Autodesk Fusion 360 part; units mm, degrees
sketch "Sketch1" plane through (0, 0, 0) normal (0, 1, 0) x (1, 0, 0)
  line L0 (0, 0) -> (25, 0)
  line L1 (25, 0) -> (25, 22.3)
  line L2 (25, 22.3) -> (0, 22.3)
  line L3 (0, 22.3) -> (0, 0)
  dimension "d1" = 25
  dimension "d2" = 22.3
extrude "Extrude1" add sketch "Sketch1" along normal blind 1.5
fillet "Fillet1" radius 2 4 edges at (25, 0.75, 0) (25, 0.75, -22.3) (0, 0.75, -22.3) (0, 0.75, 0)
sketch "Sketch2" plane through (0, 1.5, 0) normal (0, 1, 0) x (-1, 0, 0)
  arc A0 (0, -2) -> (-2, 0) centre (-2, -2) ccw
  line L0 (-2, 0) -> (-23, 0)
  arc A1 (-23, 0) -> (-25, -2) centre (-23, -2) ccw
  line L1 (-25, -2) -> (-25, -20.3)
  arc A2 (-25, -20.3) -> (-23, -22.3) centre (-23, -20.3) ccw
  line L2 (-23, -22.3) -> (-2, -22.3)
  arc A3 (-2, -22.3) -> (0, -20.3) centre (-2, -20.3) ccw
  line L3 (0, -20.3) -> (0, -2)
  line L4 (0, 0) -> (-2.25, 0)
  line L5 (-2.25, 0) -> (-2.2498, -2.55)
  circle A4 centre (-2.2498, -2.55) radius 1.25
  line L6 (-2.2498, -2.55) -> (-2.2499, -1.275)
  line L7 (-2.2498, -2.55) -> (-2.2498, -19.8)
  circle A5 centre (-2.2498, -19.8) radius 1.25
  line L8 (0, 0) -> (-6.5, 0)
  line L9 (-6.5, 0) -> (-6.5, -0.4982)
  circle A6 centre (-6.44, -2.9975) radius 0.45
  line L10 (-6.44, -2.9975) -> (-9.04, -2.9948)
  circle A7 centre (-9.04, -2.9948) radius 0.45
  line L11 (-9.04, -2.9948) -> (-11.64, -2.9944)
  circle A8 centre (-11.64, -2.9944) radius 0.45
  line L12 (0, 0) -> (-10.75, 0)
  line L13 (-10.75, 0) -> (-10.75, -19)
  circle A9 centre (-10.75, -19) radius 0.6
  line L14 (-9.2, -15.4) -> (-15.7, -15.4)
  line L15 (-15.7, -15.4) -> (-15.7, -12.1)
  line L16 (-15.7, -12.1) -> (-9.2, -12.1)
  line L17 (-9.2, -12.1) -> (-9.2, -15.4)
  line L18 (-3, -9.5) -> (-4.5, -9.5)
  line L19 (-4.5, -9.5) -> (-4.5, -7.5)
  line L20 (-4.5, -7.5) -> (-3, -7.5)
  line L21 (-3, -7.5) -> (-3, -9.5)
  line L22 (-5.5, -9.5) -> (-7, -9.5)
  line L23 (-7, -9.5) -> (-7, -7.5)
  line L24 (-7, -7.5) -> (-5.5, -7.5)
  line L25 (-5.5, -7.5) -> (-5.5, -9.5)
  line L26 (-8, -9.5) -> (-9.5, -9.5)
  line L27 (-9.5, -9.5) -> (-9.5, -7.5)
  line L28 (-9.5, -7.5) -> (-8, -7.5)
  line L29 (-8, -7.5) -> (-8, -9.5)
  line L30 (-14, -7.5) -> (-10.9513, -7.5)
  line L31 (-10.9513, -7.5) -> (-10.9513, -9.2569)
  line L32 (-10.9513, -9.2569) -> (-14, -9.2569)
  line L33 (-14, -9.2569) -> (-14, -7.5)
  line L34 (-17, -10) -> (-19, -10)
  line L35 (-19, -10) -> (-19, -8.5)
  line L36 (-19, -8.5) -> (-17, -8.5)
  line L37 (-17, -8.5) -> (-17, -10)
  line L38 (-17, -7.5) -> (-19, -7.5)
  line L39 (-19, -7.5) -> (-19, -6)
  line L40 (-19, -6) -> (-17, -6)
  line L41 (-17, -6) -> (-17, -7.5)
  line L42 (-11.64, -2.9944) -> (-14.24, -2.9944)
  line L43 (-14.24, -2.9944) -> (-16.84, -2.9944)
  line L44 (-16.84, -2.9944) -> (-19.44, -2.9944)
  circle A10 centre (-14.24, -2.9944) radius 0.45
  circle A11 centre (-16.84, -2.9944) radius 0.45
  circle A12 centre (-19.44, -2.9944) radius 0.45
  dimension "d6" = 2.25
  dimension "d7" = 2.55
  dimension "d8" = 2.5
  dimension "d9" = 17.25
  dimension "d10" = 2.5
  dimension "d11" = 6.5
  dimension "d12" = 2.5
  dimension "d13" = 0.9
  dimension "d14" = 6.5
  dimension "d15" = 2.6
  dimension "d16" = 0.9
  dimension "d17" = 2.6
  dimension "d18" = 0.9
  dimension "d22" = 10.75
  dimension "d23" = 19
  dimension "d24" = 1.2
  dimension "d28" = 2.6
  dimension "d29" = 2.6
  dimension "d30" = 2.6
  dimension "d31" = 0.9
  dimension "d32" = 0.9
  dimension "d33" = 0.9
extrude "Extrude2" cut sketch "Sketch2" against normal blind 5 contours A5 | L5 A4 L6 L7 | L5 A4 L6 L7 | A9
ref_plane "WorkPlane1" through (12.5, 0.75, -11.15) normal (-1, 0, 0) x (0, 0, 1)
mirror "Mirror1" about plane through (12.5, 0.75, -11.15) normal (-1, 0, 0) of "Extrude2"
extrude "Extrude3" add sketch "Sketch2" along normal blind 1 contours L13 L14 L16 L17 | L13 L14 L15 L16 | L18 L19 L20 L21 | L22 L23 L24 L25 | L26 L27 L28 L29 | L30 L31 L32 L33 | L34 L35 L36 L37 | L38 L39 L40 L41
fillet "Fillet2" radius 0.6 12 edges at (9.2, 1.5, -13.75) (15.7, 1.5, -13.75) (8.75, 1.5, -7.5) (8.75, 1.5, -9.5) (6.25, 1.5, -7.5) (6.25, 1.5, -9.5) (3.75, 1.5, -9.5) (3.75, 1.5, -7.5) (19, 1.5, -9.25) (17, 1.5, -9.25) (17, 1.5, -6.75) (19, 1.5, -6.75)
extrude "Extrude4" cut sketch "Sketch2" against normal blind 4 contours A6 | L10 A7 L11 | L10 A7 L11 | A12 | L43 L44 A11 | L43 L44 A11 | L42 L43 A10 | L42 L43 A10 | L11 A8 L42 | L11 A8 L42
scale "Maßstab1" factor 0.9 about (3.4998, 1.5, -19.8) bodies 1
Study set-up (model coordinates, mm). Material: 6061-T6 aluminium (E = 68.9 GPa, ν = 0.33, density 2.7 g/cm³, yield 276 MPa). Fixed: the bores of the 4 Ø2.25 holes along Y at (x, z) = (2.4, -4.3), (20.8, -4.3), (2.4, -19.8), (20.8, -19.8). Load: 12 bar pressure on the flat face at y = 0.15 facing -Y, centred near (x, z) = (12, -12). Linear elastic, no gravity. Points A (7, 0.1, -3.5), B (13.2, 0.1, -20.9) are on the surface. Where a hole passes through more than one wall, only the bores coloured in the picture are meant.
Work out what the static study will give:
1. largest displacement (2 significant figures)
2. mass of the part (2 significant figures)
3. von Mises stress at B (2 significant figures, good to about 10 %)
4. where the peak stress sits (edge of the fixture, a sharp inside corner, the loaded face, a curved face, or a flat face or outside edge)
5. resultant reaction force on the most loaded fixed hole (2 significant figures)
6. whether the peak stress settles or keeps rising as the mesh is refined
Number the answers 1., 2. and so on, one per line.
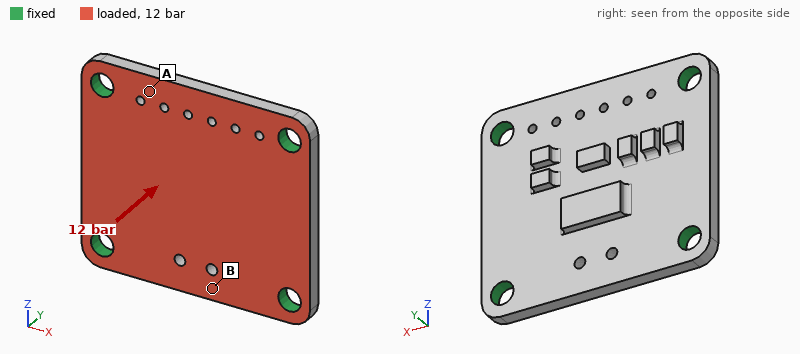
1. 33 µm
2. 1.6 g
3. 49 MPa
4. edge of the fixture
5. 130 N
6. keeps rising
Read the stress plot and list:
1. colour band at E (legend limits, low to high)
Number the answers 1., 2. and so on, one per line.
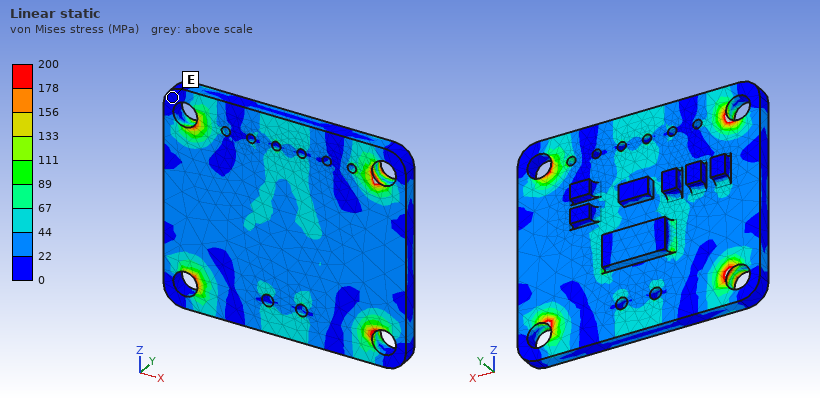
1. 0 to 22 MPa
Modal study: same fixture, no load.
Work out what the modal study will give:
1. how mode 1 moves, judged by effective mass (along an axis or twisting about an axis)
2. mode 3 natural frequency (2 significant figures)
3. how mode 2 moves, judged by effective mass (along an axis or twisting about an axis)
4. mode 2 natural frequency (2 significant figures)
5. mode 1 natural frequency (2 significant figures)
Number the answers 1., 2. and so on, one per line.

1. along Y
2. 32 kHz
3. twisting about X
4. 26 kHz
5. 18 kHz
